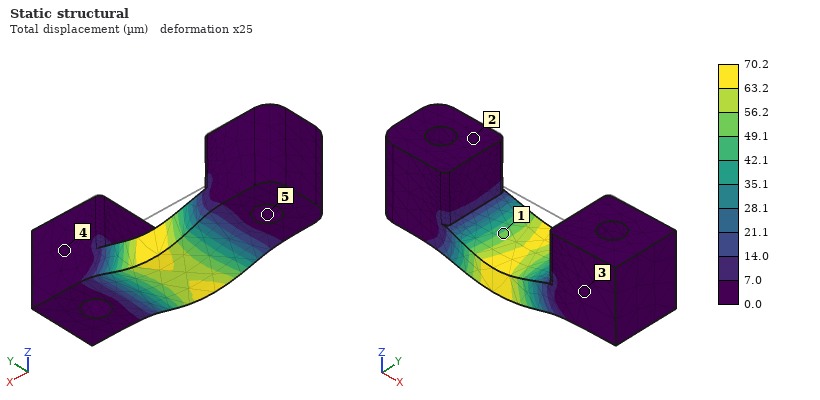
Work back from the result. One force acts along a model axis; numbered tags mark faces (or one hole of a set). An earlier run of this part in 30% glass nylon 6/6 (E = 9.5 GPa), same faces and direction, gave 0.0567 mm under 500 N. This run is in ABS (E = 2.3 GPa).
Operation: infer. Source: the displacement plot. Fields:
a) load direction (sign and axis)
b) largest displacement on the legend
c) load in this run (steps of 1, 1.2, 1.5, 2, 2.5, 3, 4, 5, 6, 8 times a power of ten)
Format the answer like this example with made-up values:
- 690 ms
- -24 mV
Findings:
- -Z
- 70.2 µm
- 150 N
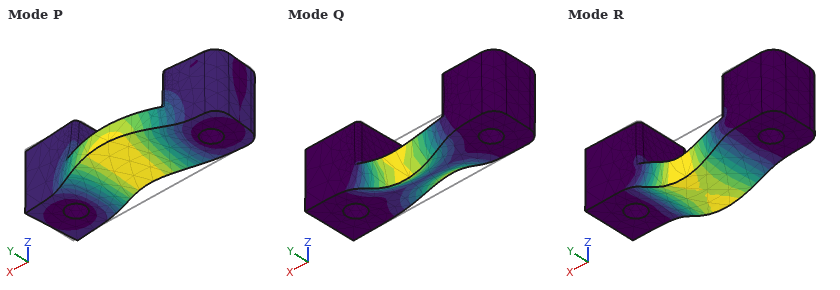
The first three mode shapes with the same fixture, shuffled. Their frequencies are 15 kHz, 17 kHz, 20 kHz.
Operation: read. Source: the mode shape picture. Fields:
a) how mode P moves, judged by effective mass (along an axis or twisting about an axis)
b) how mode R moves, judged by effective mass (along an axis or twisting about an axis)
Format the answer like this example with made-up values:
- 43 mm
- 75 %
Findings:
- along Y
- along Z
